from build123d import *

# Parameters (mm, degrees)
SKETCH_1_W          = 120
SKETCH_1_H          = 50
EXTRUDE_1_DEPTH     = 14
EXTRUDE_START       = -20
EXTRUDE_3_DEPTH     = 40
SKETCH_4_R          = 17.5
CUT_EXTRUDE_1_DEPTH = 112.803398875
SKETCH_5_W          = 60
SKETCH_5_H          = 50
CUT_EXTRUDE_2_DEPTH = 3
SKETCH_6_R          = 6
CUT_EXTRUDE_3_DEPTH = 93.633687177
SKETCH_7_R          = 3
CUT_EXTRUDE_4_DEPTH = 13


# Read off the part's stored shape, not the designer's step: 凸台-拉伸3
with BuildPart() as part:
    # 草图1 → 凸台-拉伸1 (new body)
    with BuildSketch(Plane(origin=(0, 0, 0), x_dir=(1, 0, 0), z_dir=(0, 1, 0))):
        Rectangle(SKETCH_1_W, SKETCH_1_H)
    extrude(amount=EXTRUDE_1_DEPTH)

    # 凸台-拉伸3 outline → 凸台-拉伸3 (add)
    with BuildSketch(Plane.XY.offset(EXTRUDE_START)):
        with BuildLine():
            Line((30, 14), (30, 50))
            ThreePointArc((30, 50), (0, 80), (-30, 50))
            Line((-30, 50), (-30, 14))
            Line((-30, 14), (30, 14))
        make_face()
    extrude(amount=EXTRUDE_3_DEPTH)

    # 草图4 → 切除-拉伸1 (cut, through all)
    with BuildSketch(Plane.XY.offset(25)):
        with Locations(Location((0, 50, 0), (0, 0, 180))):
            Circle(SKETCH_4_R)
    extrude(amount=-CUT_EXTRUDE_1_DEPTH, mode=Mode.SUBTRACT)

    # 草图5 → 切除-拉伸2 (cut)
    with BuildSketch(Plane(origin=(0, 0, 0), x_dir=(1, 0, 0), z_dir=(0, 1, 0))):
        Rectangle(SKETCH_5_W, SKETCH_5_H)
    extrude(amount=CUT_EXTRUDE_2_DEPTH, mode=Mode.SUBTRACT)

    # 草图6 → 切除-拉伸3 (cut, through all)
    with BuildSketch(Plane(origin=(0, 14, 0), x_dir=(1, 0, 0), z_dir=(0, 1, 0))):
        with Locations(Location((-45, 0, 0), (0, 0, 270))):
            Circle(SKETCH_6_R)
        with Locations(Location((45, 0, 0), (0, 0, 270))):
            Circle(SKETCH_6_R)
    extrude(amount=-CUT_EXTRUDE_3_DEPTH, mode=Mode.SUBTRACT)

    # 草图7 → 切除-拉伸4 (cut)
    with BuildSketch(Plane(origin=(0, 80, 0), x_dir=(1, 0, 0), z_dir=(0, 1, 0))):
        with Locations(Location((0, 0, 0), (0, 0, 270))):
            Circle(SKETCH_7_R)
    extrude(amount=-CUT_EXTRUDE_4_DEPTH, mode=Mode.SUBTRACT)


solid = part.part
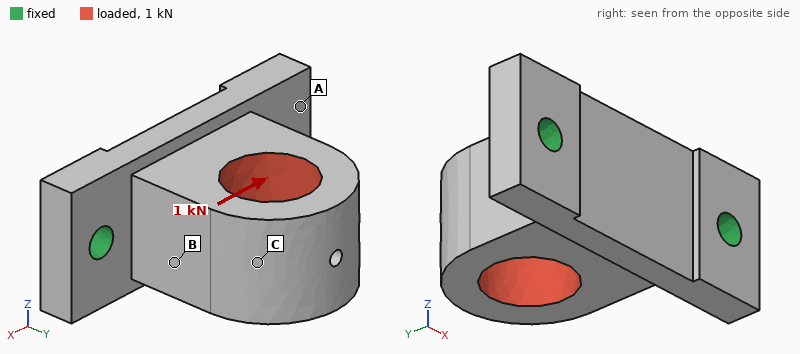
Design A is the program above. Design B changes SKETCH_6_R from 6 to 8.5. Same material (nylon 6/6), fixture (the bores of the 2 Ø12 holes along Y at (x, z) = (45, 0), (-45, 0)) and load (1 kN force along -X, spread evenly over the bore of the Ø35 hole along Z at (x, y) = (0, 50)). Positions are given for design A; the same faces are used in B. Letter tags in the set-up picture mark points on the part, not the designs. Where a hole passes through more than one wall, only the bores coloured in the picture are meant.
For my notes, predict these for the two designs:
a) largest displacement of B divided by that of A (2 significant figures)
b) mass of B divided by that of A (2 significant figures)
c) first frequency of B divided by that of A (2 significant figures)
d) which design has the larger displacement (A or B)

0.90
0.98
1.1
A
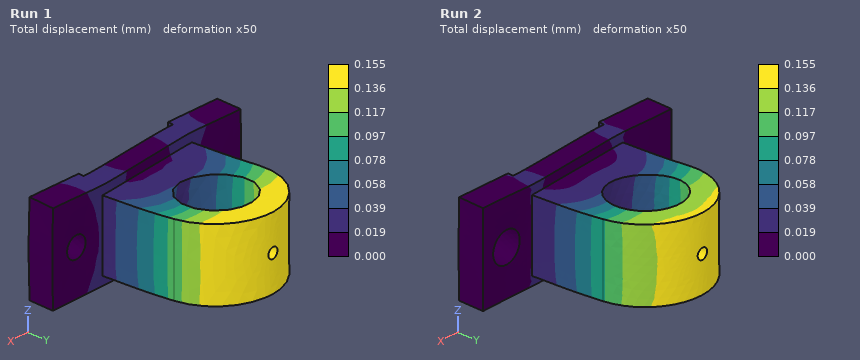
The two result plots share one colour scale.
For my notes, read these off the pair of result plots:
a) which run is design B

Run 2
